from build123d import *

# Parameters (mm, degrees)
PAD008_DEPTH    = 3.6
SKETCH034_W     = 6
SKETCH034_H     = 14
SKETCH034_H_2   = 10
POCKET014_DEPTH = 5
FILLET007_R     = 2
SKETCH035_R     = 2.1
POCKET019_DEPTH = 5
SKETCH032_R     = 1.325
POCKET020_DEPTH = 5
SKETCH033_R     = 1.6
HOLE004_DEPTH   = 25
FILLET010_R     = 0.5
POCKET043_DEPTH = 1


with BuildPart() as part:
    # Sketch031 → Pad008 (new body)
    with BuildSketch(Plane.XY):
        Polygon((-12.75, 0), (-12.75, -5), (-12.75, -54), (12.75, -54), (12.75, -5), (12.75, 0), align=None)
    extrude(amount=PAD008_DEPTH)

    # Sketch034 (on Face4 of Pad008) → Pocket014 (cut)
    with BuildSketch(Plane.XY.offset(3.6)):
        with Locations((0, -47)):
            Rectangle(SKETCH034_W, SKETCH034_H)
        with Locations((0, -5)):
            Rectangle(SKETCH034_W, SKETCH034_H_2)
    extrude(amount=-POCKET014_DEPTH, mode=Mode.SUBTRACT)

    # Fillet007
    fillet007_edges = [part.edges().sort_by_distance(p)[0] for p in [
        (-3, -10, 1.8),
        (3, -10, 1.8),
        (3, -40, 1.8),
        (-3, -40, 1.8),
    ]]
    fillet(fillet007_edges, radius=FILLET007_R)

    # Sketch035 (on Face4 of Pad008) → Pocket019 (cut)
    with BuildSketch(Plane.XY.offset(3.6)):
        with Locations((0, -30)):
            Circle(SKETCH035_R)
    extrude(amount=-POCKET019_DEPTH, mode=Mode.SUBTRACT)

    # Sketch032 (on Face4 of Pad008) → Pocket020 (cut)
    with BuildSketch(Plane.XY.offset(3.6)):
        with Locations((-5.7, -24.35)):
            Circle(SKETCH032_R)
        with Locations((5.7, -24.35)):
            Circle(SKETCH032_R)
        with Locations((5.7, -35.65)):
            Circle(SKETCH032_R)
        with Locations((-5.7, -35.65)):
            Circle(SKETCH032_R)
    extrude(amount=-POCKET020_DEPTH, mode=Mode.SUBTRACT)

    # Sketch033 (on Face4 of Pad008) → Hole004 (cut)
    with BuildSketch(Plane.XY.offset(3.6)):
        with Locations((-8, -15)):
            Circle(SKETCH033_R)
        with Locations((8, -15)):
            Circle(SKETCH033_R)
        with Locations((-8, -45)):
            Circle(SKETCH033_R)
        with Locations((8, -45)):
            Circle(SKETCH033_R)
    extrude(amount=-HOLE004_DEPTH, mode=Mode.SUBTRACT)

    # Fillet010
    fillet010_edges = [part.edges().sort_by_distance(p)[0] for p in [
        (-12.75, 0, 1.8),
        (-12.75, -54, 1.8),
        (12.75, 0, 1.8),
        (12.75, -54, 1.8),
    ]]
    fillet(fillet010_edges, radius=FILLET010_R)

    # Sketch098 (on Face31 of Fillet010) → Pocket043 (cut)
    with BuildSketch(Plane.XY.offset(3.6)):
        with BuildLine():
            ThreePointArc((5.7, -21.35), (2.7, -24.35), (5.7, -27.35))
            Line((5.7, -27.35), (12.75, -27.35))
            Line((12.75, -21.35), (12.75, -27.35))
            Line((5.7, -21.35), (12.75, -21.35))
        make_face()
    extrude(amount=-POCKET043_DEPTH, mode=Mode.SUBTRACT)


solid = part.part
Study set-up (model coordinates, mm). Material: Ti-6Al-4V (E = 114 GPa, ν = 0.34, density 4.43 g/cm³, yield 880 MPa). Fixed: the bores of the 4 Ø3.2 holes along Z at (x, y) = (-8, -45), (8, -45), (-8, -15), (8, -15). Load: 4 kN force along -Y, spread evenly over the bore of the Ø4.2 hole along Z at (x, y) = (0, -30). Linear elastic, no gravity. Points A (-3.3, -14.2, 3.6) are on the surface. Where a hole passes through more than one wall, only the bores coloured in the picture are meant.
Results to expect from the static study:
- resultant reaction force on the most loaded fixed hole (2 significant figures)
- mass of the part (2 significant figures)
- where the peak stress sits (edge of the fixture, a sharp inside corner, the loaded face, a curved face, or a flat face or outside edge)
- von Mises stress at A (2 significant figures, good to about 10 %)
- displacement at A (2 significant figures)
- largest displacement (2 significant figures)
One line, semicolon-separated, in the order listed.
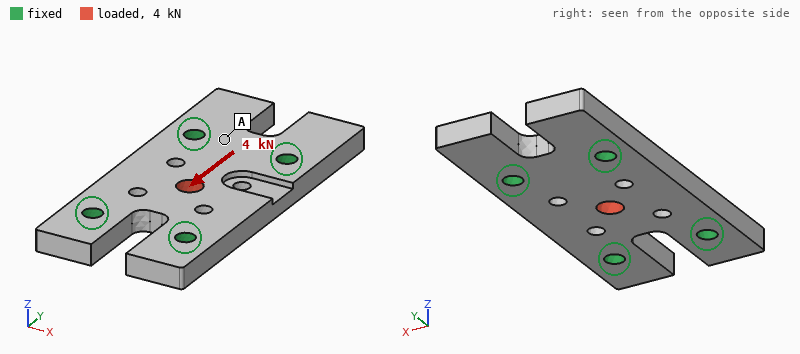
1.1 kN; 18 g; the loaded face; 16 MPa; 1.4 µm; 7.3 µm
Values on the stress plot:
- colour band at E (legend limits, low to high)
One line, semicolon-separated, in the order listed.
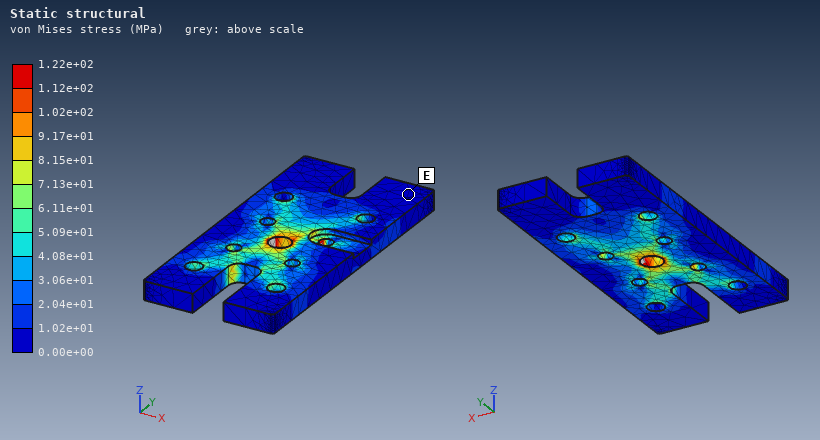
0.00e+00 to 1.02e+01 MPa
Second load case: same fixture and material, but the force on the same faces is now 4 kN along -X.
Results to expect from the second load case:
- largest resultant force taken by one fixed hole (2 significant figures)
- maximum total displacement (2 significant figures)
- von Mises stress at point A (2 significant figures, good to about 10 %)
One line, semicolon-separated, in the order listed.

1.4 kN; 14 µm; 14 MPa
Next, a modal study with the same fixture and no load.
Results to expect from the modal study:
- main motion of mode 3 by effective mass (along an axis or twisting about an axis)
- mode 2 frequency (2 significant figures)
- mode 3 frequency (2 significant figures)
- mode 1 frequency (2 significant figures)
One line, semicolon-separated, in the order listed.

along Z; 15 kHz; 19 kHz; 14 kHz
